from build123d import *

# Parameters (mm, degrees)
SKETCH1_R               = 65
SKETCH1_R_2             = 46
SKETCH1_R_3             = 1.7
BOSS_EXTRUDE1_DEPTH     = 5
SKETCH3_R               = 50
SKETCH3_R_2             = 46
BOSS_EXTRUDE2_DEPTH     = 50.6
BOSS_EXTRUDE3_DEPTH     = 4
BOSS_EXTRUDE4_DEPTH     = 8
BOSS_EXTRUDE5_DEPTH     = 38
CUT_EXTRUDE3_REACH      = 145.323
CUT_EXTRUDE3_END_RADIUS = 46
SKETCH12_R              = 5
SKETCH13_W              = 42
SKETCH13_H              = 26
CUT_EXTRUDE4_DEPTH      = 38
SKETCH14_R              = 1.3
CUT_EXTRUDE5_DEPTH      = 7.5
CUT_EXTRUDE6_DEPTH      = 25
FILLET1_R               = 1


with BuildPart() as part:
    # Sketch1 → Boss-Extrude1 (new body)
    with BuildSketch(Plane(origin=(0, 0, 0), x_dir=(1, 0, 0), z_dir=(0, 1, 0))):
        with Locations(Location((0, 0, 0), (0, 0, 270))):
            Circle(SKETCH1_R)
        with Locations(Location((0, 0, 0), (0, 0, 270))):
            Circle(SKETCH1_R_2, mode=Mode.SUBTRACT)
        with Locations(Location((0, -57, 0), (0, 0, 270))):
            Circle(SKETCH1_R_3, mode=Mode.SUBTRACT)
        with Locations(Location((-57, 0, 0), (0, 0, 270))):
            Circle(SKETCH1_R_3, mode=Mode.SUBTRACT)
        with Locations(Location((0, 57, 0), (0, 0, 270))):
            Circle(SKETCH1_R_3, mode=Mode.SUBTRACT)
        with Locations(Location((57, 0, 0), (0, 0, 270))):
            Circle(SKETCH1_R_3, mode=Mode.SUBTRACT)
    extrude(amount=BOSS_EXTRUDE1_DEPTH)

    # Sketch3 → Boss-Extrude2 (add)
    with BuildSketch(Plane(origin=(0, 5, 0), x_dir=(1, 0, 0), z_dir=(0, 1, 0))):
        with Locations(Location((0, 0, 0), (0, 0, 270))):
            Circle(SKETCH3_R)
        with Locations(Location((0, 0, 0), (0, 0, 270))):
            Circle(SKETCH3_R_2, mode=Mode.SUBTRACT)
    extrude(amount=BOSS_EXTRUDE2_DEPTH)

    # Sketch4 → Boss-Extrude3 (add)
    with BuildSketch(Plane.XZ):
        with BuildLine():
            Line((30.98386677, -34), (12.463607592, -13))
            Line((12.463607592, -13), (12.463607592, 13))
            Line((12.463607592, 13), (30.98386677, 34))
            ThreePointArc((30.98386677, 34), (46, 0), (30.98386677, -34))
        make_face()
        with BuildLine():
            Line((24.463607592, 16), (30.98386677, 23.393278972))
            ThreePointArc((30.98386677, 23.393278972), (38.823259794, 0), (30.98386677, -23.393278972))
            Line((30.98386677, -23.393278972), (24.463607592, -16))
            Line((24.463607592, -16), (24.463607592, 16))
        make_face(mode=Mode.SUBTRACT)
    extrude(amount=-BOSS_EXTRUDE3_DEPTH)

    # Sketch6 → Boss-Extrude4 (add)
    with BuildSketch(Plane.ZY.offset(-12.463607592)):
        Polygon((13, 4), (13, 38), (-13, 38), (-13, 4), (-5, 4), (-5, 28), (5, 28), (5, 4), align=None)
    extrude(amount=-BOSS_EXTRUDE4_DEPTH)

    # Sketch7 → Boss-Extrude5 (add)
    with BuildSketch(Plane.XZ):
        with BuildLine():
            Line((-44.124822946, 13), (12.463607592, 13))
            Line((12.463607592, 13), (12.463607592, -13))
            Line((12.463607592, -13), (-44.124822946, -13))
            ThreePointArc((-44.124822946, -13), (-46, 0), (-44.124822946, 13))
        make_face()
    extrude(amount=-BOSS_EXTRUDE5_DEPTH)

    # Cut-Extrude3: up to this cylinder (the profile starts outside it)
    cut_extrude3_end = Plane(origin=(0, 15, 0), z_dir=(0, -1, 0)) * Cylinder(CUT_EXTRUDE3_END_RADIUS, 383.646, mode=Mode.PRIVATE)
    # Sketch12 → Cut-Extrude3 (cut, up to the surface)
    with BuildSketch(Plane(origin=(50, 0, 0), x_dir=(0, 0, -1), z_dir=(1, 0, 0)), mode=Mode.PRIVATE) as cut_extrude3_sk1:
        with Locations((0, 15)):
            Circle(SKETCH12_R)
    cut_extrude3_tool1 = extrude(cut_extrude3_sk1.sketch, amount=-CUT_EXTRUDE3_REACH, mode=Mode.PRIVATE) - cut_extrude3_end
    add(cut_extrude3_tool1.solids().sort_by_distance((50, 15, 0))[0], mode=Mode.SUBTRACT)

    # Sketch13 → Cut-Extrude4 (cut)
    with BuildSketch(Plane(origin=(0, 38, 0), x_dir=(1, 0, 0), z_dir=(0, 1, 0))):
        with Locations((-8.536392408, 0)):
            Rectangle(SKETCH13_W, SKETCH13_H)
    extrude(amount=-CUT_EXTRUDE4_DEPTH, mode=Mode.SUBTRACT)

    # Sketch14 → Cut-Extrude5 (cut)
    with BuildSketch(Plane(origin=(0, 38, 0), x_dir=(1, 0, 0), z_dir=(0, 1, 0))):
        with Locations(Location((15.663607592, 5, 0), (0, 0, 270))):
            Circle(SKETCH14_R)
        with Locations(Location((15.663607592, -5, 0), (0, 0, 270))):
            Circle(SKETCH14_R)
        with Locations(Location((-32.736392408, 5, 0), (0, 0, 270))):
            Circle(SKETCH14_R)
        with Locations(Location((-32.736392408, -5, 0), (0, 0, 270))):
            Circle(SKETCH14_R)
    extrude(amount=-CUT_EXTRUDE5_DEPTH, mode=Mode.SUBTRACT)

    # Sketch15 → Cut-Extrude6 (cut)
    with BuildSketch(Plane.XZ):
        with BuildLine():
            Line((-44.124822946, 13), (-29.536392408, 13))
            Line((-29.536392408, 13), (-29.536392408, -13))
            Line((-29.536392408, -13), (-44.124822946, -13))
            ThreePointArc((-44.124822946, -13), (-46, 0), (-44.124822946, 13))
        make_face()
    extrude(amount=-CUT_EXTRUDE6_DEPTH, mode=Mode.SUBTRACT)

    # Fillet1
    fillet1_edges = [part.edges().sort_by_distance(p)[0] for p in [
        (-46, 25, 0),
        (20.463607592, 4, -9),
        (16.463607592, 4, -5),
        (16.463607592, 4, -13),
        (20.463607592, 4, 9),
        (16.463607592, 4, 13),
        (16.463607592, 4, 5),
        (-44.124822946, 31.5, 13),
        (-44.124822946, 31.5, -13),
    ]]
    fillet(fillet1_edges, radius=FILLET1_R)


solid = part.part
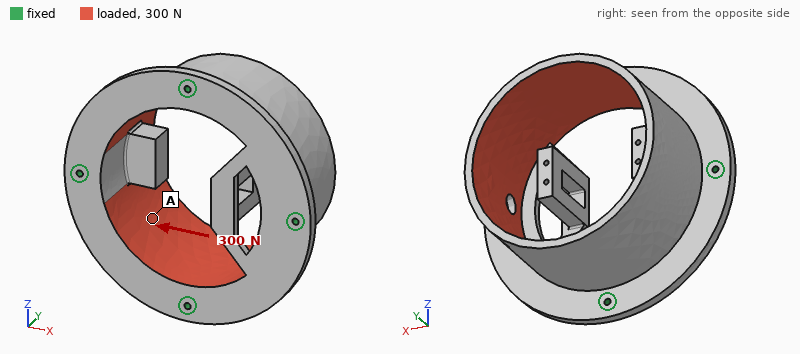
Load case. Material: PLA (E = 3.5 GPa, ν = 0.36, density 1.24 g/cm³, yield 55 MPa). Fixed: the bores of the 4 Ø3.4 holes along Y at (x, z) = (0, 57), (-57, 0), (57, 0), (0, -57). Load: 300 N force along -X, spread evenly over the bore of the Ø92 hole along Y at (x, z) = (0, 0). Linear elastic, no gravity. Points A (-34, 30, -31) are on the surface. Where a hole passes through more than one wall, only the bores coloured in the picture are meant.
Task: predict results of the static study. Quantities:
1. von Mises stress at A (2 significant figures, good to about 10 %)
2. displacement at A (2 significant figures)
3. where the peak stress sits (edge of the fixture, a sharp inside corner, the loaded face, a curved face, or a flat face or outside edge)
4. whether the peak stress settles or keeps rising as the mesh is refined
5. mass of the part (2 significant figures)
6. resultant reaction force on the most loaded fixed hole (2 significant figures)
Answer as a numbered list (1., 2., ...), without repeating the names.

1. 0.38 MPa
2. 34 µm
3. edge of the fixture
4. keeps rising
5. 130 g
6. 99 N
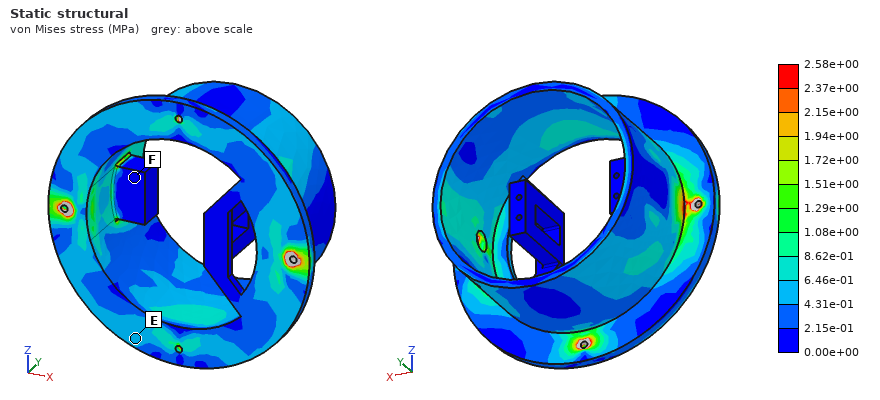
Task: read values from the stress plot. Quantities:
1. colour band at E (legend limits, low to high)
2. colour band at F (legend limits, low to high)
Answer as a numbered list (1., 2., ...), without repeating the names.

1. 4.31e-01 to 6.46e-01 MPa
2. 0.00e+00 to 2.15e-01 MPa
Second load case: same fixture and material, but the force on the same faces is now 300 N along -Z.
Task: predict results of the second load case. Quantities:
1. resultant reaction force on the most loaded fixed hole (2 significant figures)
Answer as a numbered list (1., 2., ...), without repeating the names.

1. 100 N
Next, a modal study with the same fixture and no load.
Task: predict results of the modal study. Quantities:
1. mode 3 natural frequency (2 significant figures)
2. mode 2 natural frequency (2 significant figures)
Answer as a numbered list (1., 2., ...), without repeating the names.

1. 750 Hz
2. 600 Hz
